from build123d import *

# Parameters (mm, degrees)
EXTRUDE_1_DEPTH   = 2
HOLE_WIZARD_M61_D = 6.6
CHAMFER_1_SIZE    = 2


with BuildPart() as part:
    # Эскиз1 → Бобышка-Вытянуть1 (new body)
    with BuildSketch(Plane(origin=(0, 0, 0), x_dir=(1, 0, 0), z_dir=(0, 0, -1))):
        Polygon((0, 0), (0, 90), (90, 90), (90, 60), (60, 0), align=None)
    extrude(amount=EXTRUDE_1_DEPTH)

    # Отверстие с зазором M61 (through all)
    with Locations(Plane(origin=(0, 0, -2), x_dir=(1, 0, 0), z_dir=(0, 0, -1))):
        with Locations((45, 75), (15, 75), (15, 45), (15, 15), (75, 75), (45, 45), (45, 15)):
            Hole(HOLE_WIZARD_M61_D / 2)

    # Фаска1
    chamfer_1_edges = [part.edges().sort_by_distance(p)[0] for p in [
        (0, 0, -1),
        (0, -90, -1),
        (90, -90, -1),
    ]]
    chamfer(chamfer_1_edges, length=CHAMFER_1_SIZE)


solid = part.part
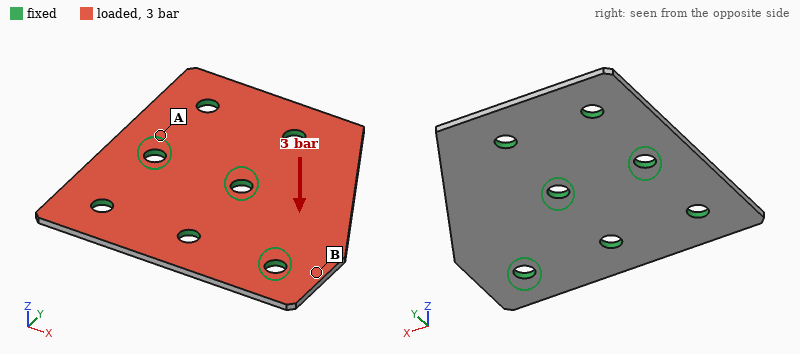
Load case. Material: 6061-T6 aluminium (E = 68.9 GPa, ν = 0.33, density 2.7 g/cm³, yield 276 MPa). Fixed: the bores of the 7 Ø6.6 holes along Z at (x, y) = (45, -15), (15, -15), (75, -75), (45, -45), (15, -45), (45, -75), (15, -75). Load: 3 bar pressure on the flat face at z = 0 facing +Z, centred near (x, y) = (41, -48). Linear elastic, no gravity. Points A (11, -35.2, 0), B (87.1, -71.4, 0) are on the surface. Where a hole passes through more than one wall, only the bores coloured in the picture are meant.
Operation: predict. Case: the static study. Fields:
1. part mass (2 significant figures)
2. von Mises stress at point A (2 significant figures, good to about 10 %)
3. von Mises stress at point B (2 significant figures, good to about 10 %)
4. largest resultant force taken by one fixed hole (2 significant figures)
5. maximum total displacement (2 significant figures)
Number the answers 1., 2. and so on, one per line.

1. 38 g
2. 16 MPa
3. 61 MPa
4. 370 N
5. 0.35 mm
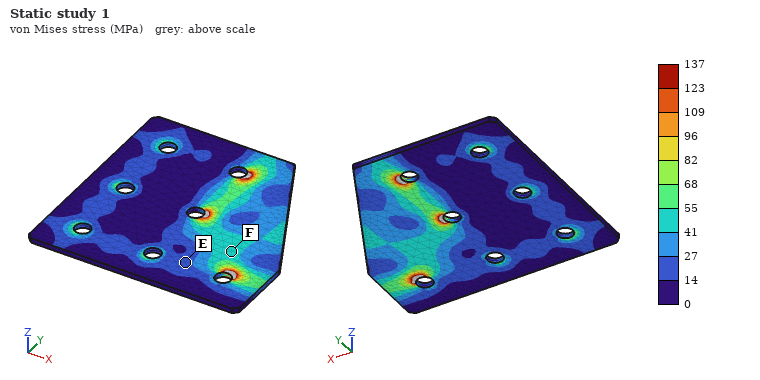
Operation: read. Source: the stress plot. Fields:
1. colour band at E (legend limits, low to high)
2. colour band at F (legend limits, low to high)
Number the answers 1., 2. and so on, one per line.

1. 14 to 27 MPa
2. 41 to 55 MPa
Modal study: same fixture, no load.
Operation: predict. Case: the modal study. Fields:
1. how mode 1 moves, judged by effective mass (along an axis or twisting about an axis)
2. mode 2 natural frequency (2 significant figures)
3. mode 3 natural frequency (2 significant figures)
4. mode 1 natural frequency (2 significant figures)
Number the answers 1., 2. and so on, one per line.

1. along Z
2. 5100 Hz
3. 7000 Hz
4. 2700 Hz
